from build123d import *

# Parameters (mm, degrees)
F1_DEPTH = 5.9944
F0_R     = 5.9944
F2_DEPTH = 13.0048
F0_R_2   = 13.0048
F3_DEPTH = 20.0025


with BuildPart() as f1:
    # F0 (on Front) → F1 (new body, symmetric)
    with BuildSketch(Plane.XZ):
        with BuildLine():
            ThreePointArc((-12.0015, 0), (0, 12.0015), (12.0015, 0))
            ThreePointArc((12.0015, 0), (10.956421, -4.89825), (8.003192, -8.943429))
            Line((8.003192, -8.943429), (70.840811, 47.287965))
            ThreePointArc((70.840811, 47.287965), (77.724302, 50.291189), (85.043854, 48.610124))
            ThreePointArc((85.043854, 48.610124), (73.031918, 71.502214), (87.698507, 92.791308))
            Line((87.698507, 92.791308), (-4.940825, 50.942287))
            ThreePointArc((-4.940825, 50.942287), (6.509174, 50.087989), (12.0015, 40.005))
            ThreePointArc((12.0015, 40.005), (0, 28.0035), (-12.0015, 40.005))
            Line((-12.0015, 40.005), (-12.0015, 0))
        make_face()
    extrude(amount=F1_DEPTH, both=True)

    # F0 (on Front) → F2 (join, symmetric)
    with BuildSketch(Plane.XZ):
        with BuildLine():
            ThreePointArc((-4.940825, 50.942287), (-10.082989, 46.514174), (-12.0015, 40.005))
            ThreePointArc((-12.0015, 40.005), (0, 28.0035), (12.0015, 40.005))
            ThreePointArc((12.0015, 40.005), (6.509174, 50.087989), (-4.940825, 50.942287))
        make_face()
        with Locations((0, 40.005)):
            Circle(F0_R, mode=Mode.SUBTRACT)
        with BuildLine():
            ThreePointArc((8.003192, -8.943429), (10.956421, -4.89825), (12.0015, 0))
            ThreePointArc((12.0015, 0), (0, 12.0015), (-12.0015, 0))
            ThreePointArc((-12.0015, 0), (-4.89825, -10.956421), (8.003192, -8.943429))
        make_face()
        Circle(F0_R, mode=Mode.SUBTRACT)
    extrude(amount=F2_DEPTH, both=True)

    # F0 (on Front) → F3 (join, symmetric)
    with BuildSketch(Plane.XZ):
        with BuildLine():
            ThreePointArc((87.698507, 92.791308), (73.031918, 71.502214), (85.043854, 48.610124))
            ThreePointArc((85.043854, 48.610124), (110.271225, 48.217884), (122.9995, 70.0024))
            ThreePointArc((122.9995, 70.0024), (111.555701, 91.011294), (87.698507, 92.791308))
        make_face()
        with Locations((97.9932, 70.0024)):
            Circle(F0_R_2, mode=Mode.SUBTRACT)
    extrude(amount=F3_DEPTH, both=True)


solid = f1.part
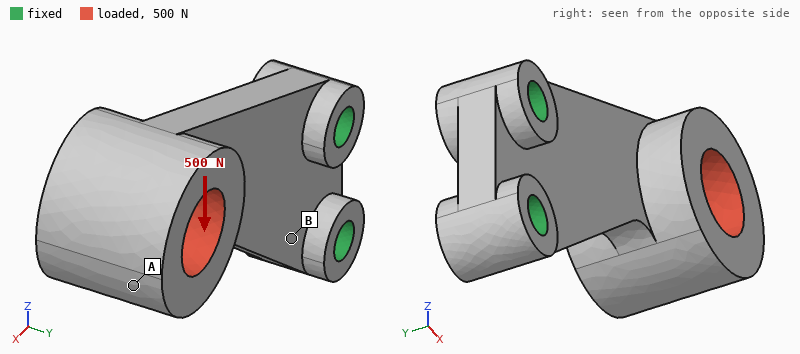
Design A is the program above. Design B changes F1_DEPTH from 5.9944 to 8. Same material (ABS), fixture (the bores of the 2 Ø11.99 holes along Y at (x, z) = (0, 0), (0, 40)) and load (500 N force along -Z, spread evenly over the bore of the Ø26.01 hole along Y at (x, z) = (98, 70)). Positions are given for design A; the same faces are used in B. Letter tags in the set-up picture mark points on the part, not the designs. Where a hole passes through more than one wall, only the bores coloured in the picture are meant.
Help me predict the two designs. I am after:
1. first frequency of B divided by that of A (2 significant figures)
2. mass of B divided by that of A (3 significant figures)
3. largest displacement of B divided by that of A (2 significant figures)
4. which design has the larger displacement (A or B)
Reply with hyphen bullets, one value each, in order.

- 1.5
- 1.13
- 0.77
- A
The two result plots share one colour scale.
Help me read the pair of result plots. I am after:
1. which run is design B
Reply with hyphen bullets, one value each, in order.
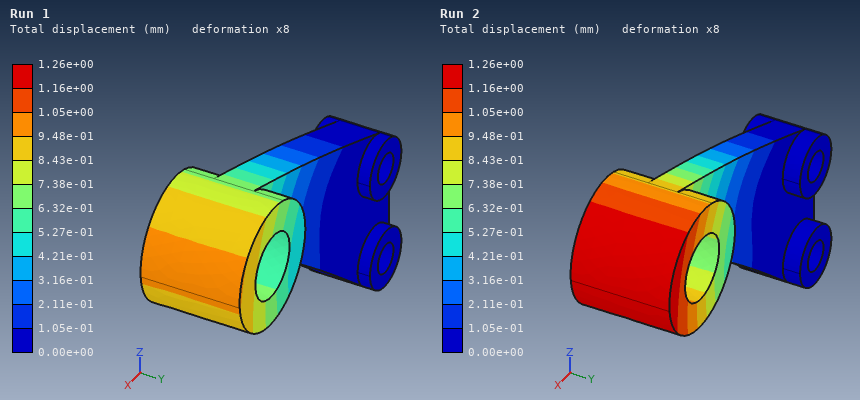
- Run 1
